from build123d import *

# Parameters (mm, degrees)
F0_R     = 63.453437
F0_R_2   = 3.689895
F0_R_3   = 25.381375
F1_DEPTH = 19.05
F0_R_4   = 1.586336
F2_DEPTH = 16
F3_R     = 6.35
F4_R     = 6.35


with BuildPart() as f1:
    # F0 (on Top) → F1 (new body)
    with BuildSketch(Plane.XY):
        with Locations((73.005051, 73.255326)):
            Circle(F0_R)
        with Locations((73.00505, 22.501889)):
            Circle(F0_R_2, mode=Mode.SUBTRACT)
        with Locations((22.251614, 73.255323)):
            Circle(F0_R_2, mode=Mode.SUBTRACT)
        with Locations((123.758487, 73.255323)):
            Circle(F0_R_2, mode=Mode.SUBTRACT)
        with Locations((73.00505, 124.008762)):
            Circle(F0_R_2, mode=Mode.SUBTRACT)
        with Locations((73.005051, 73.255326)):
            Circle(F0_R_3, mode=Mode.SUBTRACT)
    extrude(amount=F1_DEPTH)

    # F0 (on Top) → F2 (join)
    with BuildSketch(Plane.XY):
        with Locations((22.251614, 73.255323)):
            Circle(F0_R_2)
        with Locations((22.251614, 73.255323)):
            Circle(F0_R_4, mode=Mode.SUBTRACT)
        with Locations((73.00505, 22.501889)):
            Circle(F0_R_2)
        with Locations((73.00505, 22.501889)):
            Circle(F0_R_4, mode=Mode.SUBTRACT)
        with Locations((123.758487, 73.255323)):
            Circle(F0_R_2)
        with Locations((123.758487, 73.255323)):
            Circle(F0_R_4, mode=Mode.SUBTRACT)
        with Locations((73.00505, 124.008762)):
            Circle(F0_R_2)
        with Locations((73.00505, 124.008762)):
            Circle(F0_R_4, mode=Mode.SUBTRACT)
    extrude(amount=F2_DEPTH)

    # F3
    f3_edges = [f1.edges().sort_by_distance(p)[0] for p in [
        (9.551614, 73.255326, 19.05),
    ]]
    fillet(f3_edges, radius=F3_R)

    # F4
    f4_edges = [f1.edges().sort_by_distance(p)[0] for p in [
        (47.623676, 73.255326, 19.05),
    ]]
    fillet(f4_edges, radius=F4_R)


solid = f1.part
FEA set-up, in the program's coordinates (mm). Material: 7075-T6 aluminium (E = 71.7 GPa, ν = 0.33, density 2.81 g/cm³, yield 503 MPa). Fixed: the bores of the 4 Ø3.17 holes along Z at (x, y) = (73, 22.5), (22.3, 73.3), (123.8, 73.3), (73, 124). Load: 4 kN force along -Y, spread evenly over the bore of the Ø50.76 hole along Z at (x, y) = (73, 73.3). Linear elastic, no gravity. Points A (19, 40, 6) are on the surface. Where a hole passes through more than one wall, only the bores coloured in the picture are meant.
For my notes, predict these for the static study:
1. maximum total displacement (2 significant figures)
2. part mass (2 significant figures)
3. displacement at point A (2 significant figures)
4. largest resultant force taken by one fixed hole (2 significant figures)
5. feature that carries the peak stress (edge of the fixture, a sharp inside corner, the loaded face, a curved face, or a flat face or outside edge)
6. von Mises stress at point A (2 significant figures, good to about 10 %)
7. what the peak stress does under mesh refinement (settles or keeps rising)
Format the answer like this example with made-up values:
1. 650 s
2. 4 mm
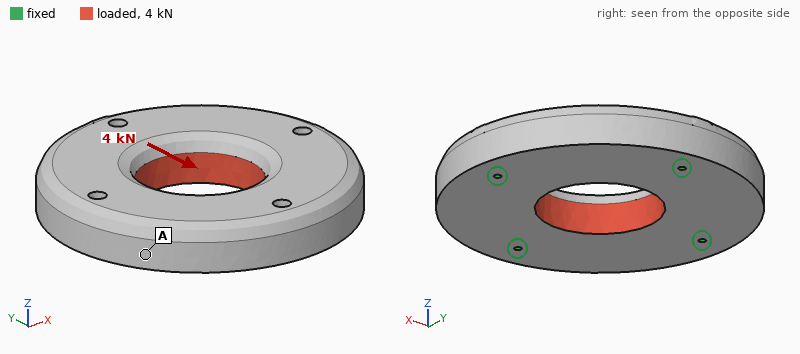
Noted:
1. 1.6 µm
2. 550 g
3. 0.77 µm
4. 1.1 kN
5. edge of the fixture
6. 1.0 MPa
7. keeps rising
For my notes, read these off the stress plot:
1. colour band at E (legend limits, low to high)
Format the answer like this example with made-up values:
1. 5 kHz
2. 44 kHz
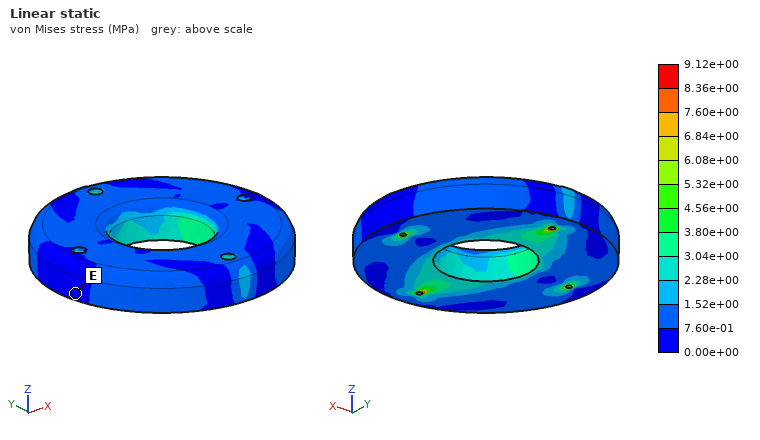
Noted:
1. 0.00e+00 to 7.60e-01 MPa
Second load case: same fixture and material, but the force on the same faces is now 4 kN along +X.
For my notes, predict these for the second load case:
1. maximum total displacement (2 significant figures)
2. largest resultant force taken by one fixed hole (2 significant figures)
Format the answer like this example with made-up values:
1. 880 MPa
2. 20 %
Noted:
1. 1.6 µm
2. 1.1 kN
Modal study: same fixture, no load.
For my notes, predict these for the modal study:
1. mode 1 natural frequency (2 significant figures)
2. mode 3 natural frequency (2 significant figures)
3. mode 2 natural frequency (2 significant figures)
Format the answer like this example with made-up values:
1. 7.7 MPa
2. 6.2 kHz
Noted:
1. 7300 Hz
2. 8800 Hz
3. 8800 Hz
